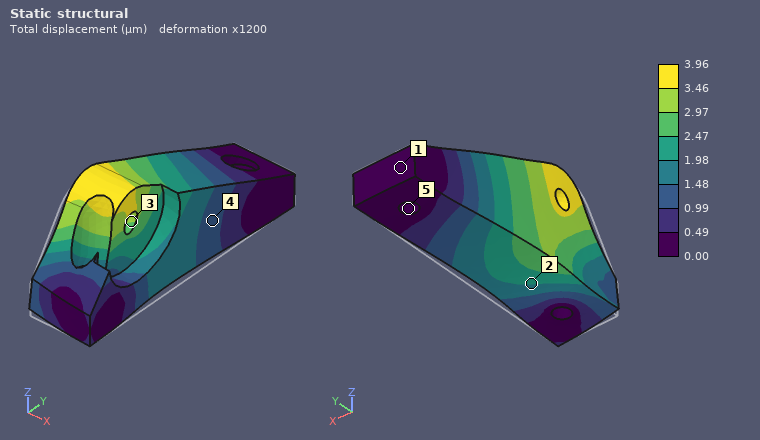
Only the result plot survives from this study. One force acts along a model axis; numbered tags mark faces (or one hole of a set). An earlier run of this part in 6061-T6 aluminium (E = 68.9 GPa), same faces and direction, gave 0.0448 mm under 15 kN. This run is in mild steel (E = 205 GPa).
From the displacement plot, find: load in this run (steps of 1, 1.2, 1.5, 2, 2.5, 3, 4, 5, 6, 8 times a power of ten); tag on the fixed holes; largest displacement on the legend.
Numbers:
4 kN
5
3.96 µm
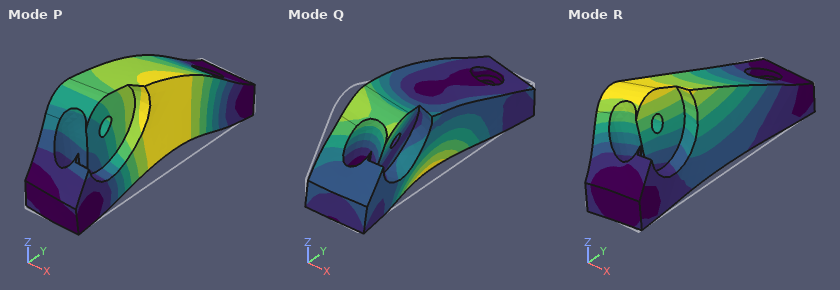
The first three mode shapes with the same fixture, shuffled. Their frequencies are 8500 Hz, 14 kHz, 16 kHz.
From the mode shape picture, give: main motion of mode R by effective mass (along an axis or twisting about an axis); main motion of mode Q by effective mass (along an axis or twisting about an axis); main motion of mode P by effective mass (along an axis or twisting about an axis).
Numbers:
along X
along X
along Z
